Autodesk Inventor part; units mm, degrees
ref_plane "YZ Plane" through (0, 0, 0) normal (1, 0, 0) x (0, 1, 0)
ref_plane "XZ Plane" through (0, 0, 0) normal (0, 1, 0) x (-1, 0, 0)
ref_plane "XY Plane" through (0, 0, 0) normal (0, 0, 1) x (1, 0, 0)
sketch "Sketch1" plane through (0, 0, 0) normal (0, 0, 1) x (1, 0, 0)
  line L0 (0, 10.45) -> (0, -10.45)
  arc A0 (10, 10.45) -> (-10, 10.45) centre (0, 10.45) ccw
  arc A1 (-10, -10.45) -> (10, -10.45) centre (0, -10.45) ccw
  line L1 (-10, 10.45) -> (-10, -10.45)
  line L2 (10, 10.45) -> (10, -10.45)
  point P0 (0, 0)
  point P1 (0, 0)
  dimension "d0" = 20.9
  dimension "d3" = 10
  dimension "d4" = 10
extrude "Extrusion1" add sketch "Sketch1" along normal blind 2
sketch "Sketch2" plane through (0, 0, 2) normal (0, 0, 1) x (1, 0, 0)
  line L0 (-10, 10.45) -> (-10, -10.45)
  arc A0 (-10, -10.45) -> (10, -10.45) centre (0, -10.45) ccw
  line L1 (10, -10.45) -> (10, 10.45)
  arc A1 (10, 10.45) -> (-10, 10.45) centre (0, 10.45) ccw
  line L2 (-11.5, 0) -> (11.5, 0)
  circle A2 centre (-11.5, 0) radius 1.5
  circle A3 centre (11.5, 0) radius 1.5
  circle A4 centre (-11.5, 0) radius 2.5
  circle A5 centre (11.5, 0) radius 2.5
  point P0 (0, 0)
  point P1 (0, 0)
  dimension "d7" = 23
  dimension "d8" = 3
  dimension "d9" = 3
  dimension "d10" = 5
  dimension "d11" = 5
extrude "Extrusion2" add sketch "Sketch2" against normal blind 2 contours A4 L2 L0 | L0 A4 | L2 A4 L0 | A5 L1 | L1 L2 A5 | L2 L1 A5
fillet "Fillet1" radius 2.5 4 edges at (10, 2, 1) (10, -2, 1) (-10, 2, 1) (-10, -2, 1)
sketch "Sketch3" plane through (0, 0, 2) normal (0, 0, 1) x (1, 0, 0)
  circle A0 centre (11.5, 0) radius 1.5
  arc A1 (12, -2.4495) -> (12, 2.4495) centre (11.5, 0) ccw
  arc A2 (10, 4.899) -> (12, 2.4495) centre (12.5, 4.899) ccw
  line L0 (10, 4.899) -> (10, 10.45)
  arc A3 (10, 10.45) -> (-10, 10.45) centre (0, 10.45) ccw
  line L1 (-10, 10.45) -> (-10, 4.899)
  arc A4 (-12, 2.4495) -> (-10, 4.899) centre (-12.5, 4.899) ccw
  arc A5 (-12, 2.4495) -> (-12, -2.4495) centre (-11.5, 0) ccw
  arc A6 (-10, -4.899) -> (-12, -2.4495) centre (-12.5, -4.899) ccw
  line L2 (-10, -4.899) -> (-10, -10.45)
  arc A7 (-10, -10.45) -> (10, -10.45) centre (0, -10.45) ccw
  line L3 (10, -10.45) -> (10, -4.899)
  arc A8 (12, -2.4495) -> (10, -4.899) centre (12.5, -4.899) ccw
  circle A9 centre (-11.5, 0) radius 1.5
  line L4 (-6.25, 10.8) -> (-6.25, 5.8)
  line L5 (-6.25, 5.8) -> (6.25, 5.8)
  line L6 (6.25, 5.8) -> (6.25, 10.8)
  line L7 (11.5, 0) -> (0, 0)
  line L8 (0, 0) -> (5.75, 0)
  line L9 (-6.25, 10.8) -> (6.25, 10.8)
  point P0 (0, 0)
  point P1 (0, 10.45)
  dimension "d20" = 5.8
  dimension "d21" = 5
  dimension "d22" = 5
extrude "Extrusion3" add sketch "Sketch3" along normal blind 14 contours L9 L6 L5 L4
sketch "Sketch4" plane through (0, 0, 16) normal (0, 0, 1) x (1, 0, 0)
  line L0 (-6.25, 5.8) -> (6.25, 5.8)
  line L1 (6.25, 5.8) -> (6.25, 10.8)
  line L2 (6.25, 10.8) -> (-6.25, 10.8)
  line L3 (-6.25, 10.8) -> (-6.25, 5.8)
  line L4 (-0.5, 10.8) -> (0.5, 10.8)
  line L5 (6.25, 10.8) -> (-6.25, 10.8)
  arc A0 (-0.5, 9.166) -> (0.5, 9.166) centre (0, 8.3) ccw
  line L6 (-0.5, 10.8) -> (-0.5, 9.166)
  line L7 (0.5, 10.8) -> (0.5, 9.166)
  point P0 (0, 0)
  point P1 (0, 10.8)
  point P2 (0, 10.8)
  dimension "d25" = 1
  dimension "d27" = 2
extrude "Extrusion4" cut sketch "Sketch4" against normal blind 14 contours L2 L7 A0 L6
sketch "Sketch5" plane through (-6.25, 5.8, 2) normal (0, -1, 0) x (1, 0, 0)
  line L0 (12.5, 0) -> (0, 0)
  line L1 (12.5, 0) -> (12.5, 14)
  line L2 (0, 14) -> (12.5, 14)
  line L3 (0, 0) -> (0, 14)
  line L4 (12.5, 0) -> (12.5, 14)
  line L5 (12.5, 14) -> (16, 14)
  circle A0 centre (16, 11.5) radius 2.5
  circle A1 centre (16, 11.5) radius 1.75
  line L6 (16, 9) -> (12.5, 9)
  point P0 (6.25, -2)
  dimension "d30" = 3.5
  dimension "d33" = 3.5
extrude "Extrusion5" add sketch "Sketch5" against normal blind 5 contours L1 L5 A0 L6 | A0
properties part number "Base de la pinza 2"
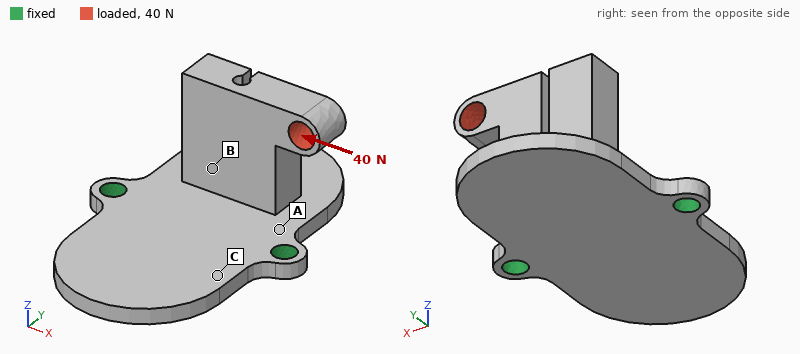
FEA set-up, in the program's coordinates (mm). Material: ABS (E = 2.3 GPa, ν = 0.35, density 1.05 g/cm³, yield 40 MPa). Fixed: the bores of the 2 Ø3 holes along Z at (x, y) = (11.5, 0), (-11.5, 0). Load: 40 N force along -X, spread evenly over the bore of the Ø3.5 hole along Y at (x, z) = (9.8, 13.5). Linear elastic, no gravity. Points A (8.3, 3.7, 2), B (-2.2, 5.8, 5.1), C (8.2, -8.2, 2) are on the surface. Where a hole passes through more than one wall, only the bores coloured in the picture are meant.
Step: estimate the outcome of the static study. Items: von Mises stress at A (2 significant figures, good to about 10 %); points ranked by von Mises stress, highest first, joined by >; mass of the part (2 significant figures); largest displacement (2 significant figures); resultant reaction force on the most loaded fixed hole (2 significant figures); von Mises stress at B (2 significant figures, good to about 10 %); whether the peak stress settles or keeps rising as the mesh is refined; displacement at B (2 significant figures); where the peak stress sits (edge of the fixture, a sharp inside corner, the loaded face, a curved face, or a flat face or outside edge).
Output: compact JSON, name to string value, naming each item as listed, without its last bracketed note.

{"von Mises stress at A": "12 MPa", "points ranked by von Mises stress, highest first, joined by >": "A > B > C", "mass of the part": "2.5 g", "largest displacement": "0.44 mm", "resultant reaction force on the most loaded fixed hole": "38 N", "von Mises stress at B": "4.9 MPa", "whether the peak stress settles or keeps rising as the mesh is refined": "keeps rising", "displacement at B": "0.11 mm", "where the peak stress sits": "edge of the fixture"}
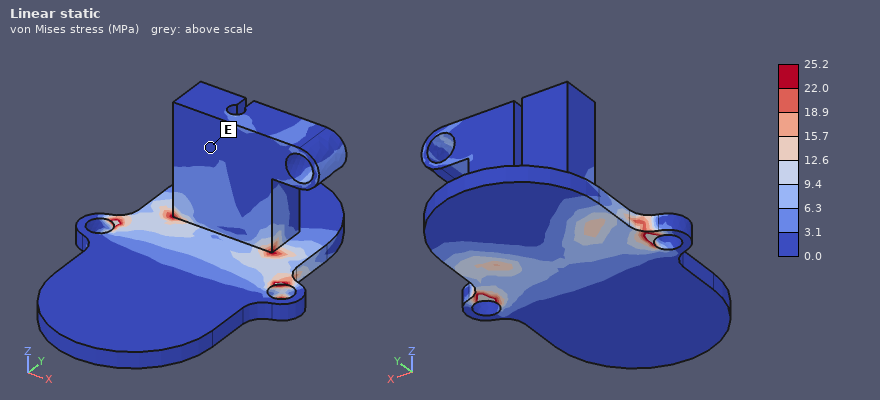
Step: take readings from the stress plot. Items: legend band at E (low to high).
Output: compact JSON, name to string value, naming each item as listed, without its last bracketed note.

{"legend band at E": "0.0 to 3.1 MPa"}
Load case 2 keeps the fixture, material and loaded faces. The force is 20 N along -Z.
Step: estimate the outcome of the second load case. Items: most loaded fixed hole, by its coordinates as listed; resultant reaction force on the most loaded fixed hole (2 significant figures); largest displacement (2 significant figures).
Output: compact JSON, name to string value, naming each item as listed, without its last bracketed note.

{"most loaded fixed hole, by its coordinates as listed": "(11.5, 0)", "resultant reaction force on the most loaded fixed hole": "21 N", "largest displacement": "0.60 mm"}
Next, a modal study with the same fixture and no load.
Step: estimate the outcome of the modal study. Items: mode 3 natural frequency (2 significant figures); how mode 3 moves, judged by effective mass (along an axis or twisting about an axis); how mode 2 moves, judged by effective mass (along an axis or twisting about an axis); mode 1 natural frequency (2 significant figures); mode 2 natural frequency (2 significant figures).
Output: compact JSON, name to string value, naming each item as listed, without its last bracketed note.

{"mode 3 natural frequency": "2200 Hz", "how mode 3 moves, judged by effective mass": "along X", "how mode 2 moves, judged by effective mass": "along Z", "mode 1 natural frequency": "740 Hz", "mode 2 natural frequency": "1300 Hz"}
